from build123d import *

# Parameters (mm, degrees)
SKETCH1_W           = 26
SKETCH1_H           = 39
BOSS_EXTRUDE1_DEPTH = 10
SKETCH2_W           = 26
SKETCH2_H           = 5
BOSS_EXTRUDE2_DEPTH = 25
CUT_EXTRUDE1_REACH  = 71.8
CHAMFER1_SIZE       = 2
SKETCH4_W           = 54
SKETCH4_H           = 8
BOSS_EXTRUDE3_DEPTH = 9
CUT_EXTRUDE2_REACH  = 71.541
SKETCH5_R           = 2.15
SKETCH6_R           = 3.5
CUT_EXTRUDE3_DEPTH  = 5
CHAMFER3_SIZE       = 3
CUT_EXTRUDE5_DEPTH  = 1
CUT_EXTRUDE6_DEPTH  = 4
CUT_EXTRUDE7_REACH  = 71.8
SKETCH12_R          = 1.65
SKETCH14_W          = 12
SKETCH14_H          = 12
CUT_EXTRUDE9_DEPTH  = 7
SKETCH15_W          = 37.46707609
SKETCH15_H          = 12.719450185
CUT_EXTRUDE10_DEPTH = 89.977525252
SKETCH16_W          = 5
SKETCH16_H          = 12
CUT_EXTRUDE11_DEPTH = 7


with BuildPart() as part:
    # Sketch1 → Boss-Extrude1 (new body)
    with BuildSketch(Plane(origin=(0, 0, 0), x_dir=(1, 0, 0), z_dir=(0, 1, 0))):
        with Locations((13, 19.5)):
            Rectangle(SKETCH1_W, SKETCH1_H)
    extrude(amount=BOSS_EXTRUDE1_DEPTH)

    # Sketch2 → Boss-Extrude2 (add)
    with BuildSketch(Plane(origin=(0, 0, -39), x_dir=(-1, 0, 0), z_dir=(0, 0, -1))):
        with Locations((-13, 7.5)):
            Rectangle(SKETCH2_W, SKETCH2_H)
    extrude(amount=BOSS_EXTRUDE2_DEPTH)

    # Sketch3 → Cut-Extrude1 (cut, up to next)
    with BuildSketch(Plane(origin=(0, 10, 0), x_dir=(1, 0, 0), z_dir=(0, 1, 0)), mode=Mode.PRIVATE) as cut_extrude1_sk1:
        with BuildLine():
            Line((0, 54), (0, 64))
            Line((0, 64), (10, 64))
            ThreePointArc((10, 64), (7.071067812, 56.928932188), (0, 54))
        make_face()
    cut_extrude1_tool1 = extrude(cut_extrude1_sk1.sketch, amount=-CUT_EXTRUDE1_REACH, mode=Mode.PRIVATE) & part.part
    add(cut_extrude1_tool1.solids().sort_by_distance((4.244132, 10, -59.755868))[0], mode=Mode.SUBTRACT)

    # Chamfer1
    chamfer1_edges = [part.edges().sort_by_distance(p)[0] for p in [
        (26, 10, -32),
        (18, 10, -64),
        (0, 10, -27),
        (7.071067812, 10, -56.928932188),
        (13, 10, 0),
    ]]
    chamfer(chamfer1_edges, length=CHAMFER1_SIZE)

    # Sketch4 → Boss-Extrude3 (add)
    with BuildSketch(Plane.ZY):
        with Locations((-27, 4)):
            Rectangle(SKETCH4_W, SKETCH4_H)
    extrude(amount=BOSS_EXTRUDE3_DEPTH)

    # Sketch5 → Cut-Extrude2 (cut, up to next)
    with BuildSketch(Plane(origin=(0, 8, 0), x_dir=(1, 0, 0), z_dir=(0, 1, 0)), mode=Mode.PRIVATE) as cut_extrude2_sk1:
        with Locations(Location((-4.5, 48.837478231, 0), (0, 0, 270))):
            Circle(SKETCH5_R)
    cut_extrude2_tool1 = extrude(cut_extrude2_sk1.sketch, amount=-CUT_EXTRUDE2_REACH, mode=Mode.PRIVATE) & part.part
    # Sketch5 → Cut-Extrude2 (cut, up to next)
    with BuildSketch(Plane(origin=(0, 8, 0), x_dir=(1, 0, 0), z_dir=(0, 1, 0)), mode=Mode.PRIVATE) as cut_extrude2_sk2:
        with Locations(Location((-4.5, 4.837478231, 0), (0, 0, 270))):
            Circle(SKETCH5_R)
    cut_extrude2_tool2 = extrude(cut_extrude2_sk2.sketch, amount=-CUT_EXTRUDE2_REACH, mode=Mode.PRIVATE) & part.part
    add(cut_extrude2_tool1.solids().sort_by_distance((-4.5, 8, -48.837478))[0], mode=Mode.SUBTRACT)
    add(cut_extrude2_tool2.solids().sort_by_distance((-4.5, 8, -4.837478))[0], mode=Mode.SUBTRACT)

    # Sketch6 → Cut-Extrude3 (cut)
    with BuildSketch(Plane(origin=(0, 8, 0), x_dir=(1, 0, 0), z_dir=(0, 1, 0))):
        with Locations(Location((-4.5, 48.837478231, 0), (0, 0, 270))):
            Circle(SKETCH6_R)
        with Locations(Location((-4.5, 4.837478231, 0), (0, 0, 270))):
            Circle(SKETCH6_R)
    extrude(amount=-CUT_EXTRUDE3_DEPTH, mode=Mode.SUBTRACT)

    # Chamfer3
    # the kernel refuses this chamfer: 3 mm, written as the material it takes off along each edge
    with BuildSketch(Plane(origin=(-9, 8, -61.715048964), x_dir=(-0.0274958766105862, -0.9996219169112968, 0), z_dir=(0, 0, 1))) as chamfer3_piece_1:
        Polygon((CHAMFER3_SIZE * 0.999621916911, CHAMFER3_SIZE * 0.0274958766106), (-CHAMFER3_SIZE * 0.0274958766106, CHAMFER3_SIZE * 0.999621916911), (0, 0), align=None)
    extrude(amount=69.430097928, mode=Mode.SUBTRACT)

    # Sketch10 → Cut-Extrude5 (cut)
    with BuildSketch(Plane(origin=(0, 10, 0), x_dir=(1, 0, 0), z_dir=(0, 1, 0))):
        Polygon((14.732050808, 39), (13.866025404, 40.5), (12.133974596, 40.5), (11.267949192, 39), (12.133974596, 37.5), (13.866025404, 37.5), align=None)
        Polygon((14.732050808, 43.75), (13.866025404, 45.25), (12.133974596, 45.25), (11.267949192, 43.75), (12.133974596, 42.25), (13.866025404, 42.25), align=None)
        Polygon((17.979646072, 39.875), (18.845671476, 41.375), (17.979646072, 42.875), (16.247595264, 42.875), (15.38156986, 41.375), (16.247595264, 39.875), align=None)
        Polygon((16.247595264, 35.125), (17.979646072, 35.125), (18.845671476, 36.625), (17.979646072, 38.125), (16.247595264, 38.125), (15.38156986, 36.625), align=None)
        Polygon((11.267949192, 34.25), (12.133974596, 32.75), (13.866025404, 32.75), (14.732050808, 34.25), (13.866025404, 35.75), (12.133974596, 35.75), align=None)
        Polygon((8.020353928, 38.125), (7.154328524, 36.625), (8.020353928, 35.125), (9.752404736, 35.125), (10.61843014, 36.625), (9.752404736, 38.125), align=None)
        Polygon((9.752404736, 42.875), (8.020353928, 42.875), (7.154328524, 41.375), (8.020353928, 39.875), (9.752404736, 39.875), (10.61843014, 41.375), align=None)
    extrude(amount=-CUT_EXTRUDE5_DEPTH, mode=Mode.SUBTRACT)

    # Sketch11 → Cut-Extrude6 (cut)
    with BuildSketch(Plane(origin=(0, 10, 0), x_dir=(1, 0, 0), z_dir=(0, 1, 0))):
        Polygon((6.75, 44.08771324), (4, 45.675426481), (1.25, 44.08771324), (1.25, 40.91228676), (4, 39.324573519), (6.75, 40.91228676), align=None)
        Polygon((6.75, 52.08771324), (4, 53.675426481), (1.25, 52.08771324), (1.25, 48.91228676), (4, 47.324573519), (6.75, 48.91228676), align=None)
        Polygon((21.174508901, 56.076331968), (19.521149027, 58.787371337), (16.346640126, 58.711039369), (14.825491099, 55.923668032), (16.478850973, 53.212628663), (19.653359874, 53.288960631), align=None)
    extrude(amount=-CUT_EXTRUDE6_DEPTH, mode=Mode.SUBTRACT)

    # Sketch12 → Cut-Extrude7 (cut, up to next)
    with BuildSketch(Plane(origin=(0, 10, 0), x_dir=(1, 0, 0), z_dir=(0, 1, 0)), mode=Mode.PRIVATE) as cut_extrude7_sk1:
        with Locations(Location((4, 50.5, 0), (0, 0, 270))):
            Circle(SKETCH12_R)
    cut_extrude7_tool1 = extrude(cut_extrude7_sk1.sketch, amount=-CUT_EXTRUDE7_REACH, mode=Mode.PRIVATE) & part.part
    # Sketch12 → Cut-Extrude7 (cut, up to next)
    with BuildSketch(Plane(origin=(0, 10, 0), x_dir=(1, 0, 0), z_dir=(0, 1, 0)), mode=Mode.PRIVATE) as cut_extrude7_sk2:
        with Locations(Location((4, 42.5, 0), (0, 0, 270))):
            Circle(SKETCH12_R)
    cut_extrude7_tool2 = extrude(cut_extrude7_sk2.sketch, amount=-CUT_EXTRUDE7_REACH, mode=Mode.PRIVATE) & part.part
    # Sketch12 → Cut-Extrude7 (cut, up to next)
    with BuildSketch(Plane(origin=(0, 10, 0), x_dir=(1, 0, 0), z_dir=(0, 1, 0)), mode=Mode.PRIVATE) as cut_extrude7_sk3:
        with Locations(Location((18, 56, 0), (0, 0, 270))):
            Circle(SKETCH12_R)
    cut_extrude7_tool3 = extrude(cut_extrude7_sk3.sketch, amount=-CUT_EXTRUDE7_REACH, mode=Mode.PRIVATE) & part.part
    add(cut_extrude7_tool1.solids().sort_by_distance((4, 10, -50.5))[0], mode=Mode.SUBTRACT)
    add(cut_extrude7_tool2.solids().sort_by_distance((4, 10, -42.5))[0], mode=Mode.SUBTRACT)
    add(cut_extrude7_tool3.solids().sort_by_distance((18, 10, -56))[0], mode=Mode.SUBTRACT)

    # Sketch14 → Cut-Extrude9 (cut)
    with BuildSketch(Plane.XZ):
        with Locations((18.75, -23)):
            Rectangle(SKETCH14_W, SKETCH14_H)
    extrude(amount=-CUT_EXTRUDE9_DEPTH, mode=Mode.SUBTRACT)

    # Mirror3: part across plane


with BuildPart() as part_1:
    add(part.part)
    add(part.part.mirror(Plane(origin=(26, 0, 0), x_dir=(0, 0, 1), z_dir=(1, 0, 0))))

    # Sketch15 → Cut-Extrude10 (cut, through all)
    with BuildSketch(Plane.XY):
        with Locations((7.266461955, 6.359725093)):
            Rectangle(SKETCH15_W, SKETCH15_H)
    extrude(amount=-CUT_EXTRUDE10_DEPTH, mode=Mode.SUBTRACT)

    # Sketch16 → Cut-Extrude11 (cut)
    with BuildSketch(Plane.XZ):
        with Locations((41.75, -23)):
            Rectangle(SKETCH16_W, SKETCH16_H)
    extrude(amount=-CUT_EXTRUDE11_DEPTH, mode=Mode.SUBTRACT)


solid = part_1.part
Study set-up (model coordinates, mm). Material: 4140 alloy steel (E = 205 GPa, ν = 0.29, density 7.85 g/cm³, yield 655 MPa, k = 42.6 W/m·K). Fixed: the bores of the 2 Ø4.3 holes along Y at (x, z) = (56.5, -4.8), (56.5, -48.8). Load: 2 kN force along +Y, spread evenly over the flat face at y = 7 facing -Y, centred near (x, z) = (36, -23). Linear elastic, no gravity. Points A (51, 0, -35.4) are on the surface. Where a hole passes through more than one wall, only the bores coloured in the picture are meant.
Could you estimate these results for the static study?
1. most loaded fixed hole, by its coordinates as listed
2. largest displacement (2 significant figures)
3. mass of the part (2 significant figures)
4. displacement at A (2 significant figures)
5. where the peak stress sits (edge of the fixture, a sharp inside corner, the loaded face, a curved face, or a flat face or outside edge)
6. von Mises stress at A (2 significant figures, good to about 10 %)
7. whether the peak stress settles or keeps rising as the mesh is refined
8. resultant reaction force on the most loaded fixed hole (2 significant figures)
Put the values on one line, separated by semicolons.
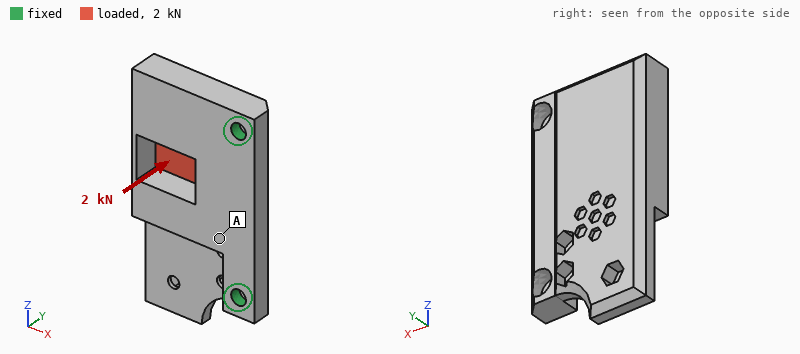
(56.5, -4.8); 0.17 mm; 110 g; 0.032 mm; edge of the fixture; 69 MPa; keeps rising; 1.4 kN
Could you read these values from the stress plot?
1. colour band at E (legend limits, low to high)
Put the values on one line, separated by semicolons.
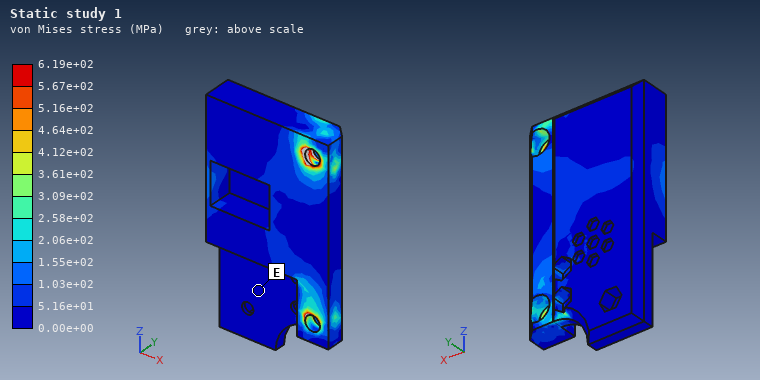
0.00e+00 to 5.16e+01 MPa
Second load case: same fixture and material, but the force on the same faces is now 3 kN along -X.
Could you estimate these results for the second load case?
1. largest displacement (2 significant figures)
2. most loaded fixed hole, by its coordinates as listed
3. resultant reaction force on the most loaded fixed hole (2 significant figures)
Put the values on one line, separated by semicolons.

54 µm; (56.5, -4.8); 1.8 kN
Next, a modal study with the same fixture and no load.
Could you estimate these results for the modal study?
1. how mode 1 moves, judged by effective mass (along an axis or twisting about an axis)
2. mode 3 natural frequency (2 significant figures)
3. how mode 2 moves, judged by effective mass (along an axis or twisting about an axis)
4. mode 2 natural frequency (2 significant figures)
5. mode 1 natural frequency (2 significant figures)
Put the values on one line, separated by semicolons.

along Y; 9800 Hz; twisting about X; 5600 Hz; 2500 Hz
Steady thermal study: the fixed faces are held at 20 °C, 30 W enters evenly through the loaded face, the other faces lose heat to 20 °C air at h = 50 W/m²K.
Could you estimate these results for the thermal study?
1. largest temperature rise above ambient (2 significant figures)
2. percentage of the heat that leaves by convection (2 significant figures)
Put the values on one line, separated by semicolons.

80 K; 36 %
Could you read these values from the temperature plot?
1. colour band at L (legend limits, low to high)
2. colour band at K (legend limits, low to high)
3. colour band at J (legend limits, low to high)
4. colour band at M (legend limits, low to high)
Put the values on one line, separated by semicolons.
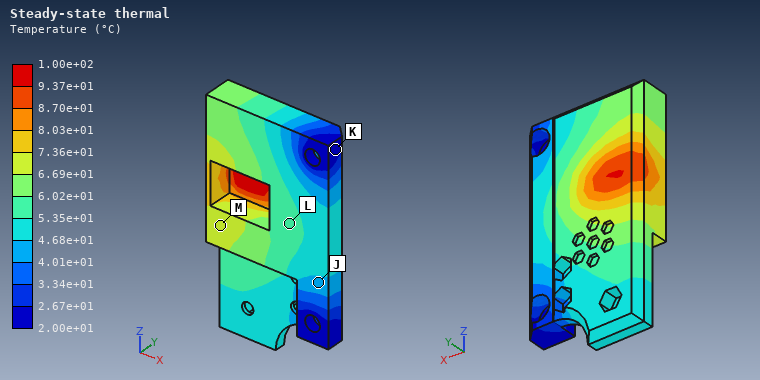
5.35e+01 to 6.02e+01 °C; 2.00e+01 to 2.67e+01 °C; 4.01e+01 to 4.68e+01 °C; 6.69e+01 to 7.36e+01 °C
